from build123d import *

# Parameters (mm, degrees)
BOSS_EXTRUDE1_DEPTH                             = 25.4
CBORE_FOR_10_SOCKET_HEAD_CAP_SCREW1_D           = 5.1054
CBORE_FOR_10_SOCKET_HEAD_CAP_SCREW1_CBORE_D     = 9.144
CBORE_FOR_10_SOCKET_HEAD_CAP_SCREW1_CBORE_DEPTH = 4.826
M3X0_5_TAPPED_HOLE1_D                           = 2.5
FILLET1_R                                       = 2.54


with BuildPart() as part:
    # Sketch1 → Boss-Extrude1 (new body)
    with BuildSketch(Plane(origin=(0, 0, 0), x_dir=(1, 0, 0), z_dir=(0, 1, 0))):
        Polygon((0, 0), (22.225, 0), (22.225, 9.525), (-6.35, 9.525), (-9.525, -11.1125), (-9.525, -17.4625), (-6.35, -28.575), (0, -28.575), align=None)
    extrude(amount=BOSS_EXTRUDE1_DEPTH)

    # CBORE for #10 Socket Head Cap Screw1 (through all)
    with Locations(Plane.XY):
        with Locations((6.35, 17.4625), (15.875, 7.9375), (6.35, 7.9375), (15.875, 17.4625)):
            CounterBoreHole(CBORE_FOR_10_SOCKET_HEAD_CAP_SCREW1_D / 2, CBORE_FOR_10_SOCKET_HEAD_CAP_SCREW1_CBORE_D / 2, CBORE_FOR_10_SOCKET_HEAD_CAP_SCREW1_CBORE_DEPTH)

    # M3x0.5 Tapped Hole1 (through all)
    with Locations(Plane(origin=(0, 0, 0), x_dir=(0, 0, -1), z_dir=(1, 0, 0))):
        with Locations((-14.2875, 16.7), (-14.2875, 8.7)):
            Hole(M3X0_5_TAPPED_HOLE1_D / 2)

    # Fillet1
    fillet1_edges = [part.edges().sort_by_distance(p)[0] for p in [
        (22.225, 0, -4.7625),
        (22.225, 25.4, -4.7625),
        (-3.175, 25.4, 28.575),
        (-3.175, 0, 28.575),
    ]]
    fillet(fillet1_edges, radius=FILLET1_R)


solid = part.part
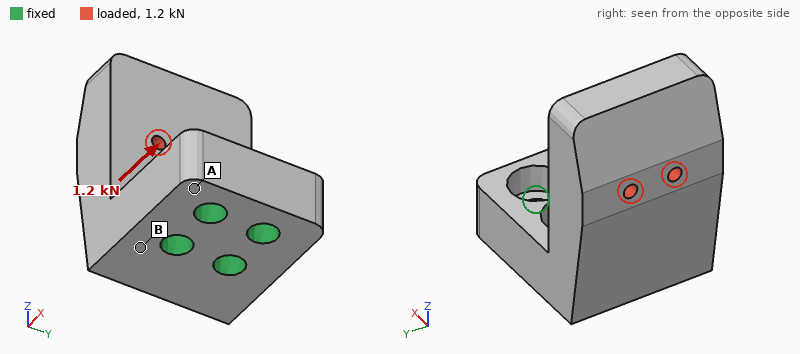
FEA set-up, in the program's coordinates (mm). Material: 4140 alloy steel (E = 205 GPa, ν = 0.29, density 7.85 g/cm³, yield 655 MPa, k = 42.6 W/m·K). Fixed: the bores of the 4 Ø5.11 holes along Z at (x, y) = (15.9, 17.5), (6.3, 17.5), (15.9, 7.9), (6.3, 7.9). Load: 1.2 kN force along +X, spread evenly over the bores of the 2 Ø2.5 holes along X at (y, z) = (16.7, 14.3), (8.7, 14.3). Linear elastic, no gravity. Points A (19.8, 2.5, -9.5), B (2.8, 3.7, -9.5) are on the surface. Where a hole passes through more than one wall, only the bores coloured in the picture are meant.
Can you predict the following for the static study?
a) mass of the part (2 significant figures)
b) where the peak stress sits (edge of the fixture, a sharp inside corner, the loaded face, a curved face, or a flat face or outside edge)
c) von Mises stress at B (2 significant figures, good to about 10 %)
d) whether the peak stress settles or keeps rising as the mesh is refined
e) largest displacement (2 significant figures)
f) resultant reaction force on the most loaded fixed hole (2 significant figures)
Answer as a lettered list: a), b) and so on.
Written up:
a) 90 g
b) a sharp inside corner
c) 76 MPa
d) keeps rising
e) 65 µm
f) 810 N
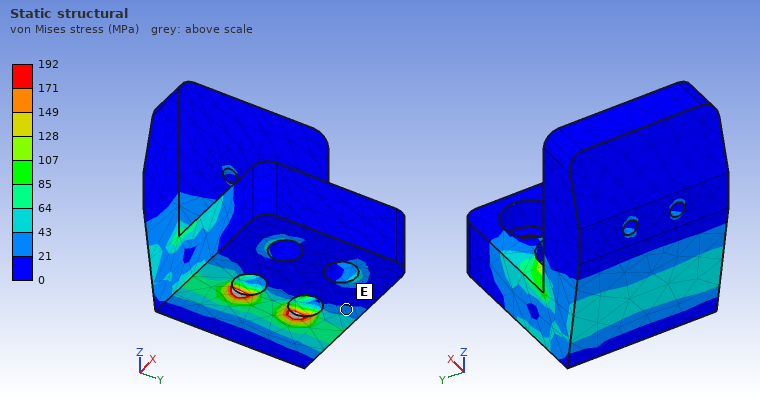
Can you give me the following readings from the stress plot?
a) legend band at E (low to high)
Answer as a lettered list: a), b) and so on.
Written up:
a) 21 to 43 MPa
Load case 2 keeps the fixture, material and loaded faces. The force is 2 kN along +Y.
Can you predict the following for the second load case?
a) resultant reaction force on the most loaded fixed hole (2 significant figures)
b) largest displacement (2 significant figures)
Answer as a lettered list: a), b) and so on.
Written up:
a) 3.1 kN
b) 41 µm
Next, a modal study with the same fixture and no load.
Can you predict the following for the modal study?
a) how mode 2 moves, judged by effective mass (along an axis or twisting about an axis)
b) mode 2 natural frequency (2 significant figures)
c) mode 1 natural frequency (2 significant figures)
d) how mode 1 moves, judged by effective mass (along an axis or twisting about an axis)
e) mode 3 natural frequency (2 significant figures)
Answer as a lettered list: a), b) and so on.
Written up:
a) along Y
b) 6000 Hz
c) 3800 Hz
d) along X
e) 14 kHz
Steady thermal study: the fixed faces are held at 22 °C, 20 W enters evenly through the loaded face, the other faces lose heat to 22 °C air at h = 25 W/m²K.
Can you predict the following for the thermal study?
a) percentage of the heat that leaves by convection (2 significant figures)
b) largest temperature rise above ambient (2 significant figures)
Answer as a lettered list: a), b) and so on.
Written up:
a) 14 %
b) 58 K
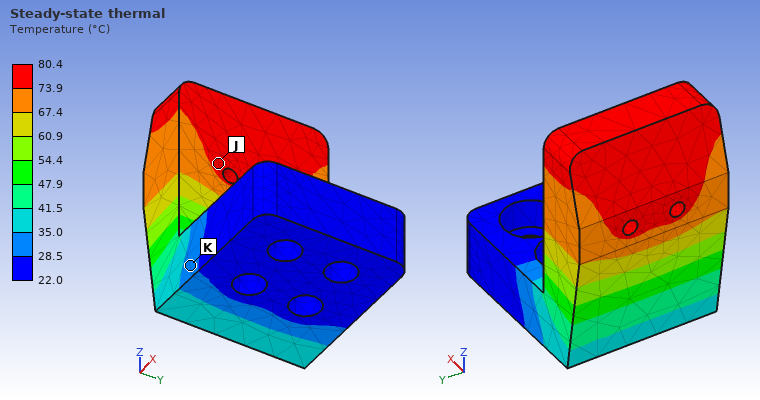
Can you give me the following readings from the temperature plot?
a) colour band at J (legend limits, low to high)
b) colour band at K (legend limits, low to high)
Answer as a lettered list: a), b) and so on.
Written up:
a) 73.9 to 80.4 °C
b) 28.5 to 35.0 °C
